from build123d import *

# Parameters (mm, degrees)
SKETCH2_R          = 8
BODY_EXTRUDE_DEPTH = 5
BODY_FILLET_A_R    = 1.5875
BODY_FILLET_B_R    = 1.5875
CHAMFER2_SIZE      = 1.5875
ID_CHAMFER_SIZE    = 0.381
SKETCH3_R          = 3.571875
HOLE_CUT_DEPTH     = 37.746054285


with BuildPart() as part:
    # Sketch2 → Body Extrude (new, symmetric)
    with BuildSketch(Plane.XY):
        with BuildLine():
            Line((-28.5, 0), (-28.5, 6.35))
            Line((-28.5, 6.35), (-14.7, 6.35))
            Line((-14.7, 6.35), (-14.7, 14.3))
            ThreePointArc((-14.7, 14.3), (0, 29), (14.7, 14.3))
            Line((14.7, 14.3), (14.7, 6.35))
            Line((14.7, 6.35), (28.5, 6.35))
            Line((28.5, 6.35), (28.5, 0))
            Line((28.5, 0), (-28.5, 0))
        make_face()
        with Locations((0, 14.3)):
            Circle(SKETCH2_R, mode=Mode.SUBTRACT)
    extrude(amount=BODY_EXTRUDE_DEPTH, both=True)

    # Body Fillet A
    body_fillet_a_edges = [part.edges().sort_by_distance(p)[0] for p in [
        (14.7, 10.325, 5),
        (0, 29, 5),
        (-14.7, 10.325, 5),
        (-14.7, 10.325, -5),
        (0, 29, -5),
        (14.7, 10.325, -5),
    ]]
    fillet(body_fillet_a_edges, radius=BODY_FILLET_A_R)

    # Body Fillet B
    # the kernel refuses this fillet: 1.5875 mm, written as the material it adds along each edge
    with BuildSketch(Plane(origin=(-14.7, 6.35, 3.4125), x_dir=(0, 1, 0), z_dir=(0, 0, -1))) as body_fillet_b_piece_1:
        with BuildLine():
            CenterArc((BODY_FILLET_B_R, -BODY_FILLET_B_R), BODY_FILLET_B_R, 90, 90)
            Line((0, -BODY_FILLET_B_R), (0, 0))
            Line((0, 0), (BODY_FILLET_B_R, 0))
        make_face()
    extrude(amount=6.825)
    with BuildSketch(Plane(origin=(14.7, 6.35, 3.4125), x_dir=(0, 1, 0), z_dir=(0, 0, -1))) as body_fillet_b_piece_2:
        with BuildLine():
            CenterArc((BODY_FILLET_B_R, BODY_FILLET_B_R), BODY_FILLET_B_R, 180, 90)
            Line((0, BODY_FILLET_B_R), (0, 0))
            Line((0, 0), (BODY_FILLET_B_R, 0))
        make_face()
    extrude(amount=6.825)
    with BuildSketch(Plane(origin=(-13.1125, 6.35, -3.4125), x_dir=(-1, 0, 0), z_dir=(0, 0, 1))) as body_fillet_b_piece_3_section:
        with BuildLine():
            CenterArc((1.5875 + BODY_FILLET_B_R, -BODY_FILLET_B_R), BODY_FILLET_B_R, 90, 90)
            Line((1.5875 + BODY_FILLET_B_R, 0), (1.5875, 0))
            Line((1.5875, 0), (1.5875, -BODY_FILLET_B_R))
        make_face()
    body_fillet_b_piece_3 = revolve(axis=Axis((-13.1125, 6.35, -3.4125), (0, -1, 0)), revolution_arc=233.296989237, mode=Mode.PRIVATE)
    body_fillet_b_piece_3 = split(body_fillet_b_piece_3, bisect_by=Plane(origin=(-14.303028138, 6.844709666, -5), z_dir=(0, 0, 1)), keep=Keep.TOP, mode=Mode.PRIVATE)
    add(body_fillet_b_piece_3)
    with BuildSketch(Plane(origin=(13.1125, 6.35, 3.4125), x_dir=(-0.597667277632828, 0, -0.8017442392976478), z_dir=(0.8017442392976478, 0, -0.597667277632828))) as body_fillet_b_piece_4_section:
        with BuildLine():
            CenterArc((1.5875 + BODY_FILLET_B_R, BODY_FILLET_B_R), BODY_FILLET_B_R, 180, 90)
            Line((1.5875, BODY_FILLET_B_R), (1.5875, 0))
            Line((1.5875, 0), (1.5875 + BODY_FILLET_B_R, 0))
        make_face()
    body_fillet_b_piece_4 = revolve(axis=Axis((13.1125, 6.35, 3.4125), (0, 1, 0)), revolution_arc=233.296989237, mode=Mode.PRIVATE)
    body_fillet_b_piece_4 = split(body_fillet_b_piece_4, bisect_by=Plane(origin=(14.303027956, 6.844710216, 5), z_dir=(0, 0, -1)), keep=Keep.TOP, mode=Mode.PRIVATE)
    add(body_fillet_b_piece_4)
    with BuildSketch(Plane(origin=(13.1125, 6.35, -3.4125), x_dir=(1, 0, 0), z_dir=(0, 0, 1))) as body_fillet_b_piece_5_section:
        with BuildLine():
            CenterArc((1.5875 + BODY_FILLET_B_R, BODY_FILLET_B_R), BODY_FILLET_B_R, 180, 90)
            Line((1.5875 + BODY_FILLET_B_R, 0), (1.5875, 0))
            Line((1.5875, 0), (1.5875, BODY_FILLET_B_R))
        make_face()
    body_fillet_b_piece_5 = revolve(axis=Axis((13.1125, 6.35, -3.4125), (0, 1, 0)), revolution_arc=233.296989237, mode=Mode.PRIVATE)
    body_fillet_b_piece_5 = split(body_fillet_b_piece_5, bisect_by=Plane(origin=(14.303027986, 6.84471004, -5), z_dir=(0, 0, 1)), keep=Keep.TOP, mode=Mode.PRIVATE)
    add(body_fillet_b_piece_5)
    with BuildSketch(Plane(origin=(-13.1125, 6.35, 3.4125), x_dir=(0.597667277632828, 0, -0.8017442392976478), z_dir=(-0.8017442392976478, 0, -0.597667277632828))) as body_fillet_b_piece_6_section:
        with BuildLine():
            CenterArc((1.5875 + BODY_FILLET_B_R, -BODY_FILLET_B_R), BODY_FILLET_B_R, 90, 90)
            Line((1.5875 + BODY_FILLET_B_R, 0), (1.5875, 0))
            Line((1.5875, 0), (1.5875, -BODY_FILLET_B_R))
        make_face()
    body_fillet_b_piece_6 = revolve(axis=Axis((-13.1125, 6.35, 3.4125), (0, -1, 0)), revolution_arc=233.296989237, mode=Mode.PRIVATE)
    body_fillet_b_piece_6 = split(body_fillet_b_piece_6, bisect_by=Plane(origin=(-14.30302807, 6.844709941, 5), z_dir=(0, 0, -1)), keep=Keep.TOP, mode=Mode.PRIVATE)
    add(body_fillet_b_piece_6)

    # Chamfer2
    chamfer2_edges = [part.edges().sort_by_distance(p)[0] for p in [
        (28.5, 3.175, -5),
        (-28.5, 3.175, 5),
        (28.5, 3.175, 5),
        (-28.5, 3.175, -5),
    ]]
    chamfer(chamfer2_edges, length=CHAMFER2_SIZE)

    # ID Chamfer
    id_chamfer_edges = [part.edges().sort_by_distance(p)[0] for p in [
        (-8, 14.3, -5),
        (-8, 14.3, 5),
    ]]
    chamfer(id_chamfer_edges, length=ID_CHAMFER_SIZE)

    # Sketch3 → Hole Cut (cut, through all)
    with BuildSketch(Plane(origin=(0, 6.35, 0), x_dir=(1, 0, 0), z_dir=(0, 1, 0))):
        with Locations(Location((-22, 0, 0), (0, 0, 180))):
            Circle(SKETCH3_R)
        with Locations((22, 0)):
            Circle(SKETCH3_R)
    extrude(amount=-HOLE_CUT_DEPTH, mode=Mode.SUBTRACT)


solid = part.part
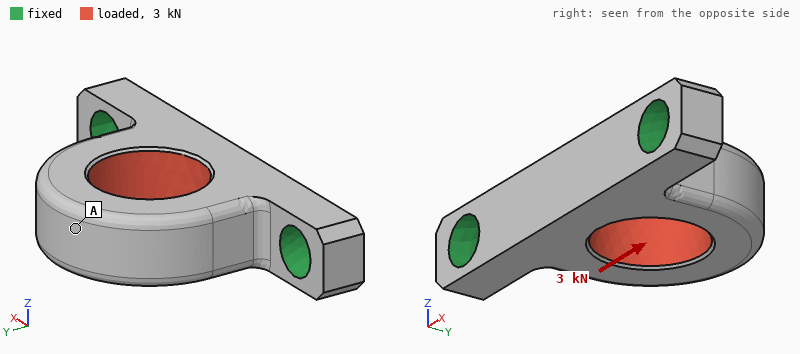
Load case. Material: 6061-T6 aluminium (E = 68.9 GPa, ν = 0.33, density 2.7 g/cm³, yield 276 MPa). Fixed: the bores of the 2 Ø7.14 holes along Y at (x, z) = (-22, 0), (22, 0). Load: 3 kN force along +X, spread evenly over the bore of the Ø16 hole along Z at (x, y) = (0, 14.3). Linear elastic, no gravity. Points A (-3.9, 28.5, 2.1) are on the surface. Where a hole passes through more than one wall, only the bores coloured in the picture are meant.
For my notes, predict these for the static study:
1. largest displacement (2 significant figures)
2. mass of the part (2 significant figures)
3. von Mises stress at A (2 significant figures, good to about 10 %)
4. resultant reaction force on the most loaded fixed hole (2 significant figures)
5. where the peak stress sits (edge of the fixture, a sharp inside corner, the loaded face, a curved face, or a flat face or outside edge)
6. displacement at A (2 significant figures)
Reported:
30 µm
18 g
13 MPa
1.8 kN
a curved face
28 µm
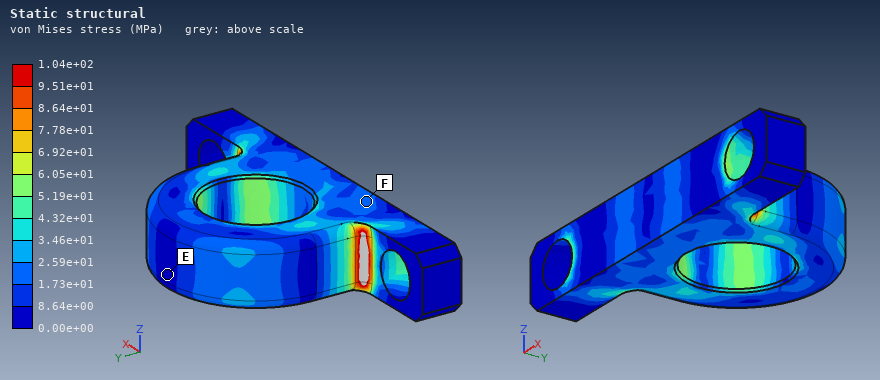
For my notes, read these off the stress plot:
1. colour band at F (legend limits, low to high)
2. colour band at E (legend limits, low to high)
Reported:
1.73e+01 to 2.59e+01 MPa
0.00e+00 to 8.64e+00 MPa
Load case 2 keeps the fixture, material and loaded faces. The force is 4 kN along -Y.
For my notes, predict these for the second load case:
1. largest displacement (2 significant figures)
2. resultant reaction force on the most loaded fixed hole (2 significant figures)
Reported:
28 µm
2.1 kN
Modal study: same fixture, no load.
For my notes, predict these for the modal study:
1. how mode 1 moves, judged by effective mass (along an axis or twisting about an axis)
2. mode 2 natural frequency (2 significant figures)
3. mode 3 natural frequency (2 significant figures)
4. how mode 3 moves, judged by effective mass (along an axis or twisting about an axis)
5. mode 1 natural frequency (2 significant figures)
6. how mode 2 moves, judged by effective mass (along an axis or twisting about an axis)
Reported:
along Z
16 kHz
18 kHz
twisting about Y
6000 Hz
along X
